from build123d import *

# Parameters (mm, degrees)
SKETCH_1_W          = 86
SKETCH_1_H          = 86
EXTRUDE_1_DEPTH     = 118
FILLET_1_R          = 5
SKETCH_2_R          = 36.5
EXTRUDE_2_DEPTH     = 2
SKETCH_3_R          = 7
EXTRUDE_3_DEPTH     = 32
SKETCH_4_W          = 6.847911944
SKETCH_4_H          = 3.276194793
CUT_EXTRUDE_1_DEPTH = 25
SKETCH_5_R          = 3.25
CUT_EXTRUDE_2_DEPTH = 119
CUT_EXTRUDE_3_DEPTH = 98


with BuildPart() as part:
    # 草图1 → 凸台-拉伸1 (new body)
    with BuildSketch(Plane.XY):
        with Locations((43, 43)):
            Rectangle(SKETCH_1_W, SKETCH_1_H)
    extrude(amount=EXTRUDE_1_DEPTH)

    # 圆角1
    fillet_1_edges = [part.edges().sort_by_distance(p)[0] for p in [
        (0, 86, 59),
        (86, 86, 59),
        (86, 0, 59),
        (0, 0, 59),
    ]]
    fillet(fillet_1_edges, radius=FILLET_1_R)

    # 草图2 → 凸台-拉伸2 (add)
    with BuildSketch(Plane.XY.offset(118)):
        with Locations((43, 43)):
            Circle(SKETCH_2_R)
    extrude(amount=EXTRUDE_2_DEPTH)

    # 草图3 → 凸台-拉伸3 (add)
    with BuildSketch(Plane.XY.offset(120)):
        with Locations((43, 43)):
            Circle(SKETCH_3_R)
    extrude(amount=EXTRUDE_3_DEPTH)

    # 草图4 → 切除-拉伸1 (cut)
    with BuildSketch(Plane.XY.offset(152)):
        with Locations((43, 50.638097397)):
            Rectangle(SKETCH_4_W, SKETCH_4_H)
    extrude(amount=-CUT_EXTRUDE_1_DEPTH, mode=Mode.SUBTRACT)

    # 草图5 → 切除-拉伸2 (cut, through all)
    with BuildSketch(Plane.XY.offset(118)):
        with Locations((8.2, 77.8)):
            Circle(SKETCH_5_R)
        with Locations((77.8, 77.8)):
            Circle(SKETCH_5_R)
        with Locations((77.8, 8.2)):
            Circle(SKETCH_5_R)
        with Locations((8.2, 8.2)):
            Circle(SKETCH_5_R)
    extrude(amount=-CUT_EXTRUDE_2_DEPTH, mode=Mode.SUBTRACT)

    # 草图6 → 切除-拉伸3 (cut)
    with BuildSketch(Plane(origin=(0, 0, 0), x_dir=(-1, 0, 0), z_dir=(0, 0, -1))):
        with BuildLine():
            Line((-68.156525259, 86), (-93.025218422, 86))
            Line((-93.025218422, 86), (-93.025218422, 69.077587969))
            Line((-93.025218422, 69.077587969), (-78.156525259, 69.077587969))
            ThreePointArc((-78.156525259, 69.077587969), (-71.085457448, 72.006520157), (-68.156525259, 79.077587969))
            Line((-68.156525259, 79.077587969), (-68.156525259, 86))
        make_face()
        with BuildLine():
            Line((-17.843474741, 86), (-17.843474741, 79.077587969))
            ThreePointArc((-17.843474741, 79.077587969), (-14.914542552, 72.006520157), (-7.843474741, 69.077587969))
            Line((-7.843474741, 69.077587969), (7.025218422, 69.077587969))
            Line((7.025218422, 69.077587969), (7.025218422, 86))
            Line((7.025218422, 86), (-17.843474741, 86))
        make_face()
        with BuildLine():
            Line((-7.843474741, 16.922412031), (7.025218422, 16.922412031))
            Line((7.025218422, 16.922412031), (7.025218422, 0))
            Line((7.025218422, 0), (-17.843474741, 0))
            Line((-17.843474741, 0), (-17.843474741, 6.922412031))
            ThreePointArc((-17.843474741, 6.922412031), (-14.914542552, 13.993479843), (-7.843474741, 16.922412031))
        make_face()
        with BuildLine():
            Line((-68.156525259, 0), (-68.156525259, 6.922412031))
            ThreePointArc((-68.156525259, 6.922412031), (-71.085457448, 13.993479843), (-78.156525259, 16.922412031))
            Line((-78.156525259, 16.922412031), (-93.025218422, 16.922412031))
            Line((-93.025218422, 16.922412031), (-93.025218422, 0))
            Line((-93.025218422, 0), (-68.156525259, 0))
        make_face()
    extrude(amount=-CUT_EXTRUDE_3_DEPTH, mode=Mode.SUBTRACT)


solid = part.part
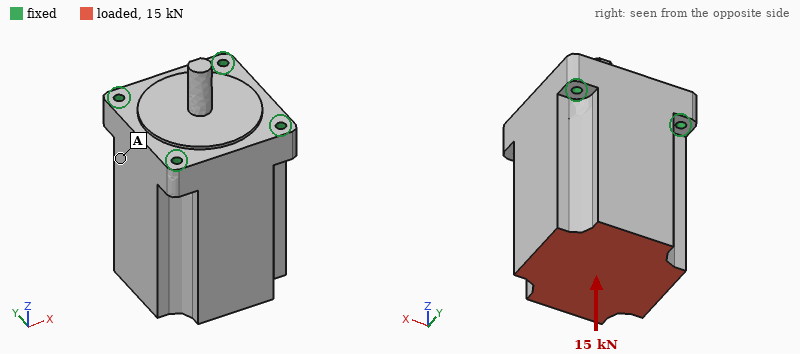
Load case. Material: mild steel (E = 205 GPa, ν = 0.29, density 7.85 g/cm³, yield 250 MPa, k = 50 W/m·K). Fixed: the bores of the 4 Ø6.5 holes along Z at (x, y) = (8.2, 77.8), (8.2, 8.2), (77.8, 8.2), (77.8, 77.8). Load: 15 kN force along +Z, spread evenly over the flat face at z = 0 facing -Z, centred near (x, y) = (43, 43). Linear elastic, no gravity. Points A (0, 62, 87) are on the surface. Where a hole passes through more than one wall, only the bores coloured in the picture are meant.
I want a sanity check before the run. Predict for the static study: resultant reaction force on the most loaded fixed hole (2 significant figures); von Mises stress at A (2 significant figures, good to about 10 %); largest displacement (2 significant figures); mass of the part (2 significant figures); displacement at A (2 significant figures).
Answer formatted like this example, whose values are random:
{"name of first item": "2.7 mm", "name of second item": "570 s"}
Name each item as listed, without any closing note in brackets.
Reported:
{"resultant reaction force on the most loaded fixed hole": "3.9 kN", "von Mises stress at A": "4.8 MPa", "largest displacement": "2.7 µm", "mass of the part": "6.1 kg", "displacement at A": "1.6 µm"}
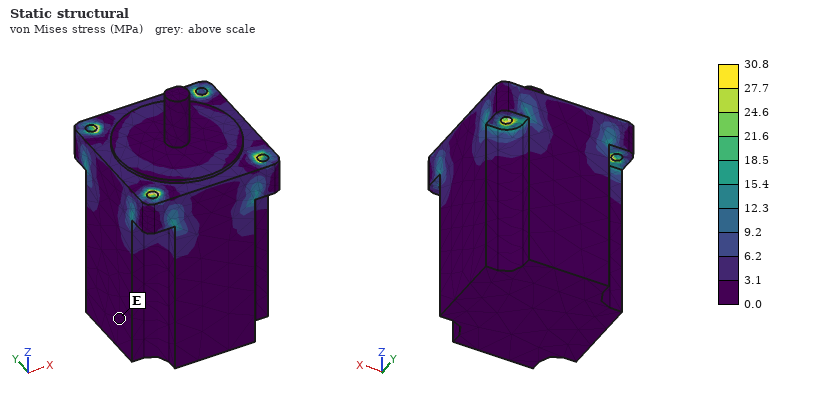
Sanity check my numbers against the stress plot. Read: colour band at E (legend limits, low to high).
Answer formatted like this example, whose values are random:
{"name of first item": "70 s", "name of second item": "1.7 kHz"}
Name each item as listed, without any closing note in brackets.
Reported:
{"colour band at E": "0.0 to 3.1 MPa"}
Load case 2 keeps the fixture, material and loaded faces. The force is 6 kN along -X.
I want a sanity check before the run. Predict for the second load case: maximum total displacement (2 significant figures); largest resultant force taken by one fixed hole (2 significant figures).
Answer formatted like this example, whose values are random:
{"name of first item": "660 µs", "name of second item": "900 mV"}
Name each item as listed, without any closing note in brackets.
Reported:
{"maximum total displacement": "12 µm", "largest resultant force taken by one fixed hole": "5.0 kN"}
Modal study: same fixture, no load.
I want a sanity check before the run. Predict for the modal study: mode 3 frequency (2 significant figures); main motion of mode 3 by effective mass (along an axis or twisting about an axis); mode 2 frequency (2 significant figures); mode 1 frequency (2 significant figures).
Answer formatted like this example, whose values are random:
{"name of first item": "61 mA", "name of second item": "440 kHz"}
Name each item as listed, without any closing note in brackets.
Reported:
{"mode 3 frequency": "5900 Hz", "main motion of mode 3 by effective mass": "along Z", "mode 2 frequency": "2800 Hz", "mode 1 frequency": "2800 Hz"}
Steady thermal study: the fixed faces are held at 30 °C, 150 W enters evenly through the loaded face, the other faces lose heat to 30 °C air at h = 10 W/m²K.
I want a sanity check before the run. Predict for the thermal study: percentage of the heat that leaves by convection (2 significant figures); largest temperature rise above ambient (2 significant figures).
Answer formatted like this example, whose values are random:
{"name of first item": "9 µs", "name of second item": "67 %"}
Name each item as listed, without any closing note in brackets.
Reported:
{"percentage of the heat that leaves by convection": "10 %", "largest temperature rise above ambient": "64 K"}
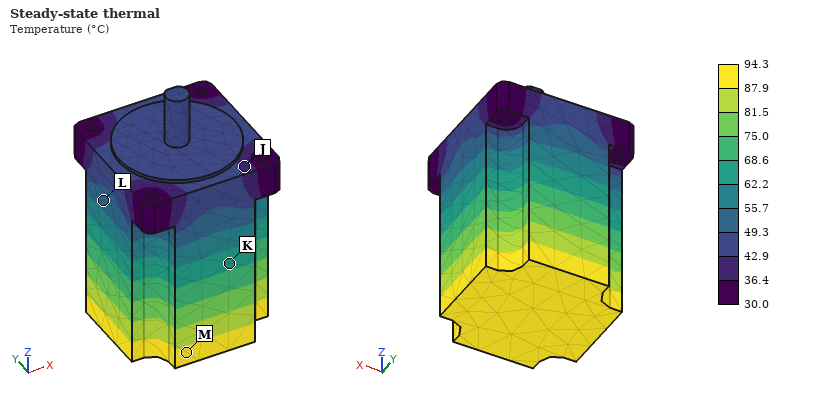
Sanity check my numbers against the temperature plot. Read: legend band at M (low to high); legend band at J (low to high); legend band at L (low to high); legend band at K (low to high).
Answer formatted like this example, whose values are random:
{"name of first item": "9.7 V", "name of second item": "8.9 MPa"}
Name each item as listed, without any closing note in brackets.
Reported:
{"legend band at M": "87.9 to 94.3 °C", "legend band at J": "36.4 to 42.9 °C", "legend band at L": "49.3 to 55.7 °C", "legend band at K": "62.2 to 68.6 °C"}
